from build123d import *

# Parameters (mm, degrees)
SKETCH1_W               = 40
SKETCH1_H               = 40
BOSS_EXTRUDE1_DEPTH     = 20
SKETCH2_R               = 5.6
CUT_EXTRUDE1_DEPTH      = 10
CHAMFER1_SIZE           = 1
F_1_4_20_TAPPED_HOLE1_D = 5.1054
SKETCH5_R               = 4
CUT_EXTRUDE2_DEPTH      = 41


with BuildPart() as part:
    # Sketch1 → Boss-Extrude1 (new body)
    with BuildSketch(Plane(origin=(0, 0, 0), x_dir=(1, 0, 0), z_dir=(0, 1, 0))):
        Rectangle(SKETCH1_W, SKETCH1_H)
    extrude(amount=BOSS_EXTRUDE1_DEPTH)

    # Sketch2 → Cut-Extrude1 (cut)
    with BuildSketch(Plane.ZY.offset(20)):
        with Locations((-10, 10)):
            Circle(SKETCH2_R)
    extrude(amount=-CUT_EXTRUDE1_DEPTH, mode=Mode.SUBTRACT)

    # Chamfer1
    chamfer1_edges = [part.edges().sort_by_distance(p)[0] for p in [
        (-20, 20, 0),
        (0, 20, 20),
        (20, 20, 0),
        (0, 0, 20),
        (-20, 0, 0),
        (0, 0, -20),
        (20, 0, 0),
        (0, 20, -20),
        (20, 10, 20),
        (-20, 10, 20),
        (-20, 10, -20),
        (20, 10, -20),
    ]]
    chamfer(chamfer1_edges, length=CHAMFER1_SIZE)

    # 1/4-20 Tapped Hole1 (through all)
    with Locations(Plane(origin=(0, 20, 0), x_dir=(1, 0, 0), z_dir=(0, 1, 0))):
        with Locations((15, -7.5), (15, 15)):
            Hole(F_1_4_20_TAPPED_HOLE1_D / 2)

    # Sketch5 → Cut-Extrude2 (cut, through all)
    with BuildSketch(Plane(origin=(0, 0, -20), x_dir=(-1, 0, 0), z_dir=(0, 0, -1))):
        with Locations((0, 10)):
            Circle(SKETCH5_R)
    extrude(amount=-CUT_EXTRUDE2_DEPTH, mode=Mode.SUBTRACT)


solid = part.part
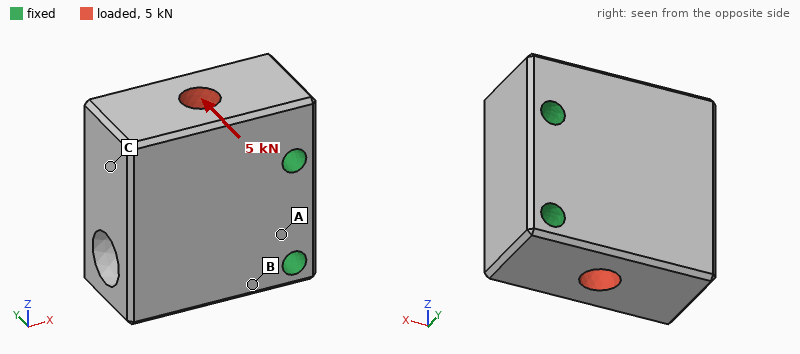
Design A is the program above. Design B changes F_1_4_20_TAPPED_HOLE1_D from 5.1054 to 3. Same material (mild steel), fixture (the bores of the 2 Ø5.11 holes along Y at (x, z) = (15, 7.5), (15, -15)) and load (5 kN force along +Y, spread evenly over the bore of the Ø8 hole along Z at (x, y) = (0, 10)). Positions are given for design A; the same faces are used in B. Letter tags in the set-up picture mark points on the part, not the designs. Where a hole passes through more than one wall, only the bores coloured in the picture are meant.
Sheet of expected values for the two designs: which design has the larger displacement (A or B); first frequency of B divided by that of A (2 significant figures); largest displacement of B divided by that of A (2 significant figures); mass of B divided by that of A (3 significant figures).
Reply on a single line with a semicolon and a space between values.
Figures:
B; 0.90; 1.3; 1.02
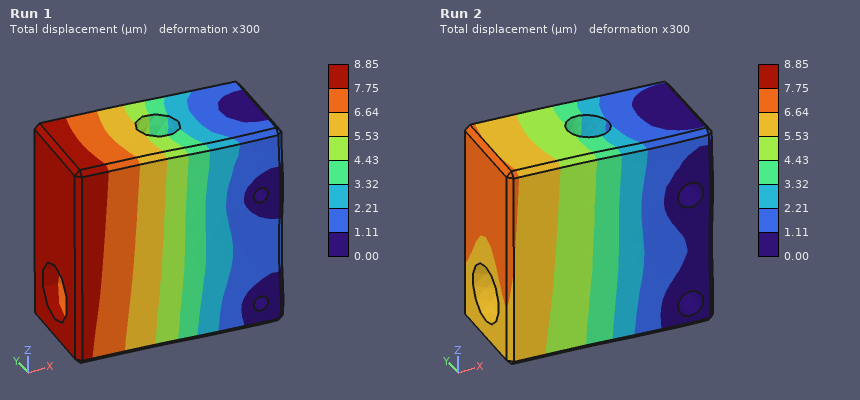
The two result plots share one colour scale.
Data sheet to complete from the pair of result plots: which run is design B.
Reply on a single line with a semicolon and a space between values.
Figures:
Run 1
